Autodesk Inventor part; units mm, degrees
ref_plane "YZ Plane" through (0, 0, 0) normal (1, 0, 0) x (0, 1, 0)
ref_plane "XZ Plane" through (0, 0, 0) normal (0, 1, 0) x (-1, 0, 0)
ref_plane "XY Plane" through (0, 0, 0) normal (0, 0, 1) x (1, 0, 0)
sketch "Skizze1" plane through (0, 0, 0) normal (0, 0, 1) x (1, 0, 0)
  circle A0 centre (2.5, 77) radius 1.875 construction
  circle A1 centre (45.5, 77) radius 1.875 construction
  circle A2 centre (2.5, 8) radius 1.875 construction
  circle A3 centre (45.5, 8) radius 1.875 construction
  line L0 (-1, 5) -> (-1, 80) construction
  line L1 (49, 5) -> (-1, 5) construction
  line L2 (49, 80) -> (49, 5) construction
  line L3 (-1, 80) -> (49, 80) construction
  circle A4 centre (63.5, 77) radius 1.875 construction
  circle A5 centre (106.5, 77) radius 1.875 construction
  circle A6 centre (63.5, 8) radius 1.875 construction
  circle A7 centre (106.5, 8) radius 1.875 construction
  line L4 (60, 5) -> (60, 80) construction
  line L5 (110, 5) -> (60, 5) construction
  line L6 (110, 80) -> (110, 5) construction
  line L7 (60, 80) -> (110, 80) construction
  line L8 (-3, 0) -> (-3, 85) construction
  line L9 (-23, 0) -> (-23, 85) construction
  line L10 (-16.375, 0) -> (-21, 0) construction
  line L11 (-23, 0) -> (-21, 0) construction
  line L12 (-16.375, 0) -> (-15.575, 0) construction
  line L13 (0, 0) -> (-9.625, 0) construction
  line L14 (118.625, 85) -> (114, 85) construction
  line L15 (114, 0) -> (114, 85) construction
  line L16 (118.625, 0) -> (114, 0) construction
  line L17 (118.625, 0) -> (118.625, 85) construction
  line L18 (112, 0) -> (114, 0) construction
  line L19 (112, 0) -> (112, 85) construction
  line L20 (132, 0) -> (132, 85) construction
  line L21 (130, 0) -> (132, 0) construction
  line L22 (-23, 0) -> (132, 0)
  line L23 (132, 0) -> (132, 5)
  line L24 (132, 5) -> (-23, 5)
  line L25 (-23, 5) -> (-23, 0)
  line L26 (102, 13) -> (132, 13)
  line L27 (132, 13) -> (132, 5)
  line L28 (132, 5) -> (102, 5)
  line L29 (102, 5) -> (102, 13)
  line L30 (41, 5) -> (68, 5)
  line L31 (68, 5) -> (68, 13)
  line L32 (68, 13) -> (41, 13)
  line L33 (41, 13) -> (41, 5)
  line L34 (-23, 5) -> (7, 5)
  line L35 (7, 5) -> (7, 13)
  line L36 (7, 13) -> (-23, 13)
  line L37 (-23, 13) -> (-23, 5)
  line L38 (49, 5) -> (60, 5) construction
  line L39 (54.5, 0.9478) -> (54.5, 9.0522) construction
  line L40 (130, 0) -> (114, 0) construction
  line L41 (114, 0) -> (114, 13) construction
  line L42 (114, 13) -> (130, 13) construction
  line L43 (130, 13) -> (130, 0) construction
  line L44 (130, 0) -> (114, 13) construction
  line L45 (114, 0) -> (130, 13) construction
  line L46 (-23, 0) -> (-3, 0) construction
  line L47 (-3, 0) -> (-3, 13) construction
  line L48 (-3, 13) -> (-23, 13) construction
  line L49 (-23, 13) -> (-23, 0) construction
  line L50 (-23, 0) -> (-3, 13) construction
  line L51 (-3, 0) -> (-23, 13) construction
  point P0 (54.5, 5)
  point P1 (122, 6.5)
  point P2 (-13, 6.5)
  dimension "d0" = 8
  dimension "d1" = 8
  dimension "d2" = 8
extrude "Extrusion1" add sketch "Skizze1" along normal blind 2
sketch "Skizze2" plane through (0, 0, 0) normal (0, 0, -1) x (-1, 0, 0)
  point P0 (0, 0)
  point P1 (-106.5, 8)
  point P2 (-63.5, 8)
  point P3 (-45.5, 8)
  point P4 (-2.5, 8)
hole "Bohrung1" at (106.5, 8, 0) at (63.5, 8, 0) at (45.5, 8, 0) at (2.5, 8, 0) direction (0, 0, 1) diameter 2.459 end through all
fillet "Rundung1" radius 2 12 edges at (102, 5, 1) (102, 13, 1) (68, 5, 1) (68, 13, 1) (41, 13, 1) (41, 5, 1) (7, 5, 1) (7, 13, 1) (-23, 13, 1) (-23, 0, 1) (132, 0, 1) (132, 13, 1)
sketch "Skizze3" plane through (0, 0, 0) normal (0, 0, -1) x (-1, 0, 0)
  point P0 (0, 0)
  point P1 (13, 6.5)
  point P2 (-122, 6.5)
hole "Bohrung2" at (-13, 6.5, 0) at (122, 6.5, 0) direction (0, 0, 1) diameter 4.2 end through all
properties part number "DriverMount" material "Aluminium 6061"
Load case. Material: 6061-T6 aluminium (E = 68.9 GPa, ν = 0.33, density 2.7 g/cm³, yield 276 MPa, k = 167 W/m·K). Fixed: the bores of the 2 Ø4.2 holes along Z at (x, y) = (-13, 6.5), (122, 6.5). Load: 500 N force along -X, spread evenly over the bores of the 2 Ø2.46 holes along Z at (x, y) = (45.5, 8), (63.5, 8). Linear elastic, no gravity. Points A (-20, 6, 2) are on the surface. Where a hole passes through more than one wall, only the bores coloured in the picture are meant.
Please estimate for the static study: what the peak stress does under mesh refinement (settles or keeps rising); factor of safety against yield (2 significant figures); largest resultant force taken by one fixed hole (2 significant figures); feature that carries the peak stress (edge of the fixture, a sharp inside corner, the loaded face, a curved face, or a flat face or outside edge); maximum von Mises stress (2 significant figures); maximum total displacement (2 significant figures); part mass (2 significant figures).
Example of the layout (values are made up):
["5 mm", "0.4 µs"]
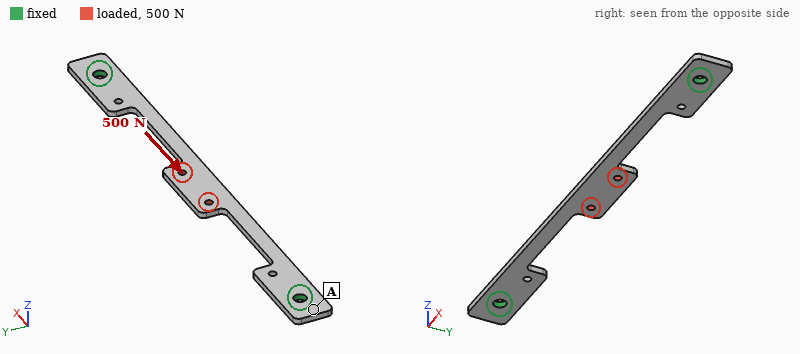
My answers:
["settles", "1.6", "250 N", "a curved face", "180 MPa", "0.10 mm", "7.7 g"]
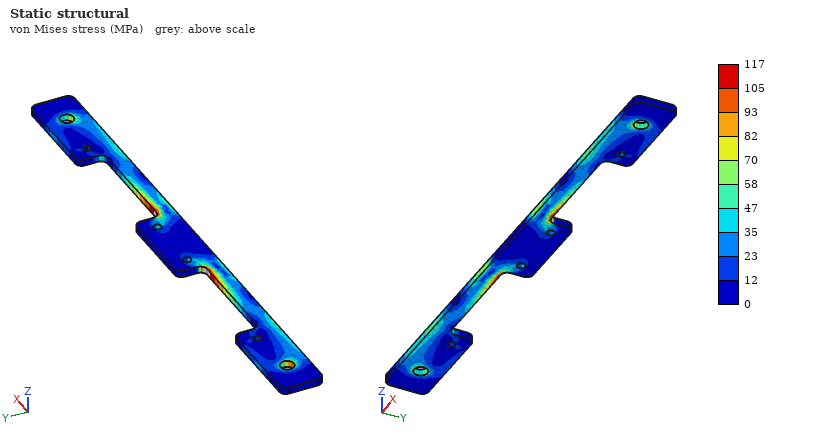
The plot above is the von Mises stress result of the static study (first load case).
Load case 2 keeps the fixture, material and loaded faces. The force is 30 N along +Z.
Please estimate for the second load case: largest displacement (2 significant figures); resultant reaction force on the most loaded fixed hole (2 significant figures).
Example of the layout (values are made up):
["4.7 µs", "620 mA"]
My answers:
["0.92 mm", "15 N"]
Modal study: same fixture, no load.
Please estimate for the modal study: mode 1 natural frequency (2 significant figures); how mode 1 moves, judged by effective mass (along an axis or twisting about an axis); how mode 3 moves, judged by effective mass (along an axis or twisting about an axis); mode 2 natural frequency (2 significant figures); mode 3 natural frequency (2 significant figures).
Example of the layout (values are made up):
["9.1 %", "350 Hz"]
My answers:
["610 Hz", "along Z", "along Y", "1800 Hz", "2100 Hz"]
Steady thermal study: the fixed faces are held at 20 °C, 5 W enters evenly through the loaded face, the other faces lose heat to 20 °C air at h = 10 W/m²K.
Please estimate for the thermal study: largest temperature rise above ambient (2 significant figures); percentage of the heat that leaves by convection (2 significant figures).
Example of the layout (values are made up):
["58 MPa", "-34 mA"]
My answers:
["62 K", "17 %"]
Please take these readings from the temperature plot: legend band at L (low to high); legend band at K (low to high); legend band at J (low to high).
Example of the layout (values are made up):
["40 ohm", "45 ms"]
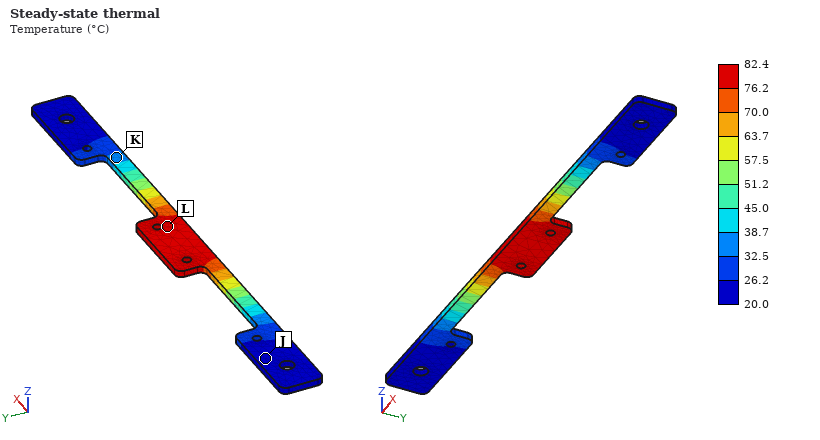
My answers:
["76.2 to 82.4 °C", "32.5 to 38.7 °C", "20.0 to 26.2 °C"]
